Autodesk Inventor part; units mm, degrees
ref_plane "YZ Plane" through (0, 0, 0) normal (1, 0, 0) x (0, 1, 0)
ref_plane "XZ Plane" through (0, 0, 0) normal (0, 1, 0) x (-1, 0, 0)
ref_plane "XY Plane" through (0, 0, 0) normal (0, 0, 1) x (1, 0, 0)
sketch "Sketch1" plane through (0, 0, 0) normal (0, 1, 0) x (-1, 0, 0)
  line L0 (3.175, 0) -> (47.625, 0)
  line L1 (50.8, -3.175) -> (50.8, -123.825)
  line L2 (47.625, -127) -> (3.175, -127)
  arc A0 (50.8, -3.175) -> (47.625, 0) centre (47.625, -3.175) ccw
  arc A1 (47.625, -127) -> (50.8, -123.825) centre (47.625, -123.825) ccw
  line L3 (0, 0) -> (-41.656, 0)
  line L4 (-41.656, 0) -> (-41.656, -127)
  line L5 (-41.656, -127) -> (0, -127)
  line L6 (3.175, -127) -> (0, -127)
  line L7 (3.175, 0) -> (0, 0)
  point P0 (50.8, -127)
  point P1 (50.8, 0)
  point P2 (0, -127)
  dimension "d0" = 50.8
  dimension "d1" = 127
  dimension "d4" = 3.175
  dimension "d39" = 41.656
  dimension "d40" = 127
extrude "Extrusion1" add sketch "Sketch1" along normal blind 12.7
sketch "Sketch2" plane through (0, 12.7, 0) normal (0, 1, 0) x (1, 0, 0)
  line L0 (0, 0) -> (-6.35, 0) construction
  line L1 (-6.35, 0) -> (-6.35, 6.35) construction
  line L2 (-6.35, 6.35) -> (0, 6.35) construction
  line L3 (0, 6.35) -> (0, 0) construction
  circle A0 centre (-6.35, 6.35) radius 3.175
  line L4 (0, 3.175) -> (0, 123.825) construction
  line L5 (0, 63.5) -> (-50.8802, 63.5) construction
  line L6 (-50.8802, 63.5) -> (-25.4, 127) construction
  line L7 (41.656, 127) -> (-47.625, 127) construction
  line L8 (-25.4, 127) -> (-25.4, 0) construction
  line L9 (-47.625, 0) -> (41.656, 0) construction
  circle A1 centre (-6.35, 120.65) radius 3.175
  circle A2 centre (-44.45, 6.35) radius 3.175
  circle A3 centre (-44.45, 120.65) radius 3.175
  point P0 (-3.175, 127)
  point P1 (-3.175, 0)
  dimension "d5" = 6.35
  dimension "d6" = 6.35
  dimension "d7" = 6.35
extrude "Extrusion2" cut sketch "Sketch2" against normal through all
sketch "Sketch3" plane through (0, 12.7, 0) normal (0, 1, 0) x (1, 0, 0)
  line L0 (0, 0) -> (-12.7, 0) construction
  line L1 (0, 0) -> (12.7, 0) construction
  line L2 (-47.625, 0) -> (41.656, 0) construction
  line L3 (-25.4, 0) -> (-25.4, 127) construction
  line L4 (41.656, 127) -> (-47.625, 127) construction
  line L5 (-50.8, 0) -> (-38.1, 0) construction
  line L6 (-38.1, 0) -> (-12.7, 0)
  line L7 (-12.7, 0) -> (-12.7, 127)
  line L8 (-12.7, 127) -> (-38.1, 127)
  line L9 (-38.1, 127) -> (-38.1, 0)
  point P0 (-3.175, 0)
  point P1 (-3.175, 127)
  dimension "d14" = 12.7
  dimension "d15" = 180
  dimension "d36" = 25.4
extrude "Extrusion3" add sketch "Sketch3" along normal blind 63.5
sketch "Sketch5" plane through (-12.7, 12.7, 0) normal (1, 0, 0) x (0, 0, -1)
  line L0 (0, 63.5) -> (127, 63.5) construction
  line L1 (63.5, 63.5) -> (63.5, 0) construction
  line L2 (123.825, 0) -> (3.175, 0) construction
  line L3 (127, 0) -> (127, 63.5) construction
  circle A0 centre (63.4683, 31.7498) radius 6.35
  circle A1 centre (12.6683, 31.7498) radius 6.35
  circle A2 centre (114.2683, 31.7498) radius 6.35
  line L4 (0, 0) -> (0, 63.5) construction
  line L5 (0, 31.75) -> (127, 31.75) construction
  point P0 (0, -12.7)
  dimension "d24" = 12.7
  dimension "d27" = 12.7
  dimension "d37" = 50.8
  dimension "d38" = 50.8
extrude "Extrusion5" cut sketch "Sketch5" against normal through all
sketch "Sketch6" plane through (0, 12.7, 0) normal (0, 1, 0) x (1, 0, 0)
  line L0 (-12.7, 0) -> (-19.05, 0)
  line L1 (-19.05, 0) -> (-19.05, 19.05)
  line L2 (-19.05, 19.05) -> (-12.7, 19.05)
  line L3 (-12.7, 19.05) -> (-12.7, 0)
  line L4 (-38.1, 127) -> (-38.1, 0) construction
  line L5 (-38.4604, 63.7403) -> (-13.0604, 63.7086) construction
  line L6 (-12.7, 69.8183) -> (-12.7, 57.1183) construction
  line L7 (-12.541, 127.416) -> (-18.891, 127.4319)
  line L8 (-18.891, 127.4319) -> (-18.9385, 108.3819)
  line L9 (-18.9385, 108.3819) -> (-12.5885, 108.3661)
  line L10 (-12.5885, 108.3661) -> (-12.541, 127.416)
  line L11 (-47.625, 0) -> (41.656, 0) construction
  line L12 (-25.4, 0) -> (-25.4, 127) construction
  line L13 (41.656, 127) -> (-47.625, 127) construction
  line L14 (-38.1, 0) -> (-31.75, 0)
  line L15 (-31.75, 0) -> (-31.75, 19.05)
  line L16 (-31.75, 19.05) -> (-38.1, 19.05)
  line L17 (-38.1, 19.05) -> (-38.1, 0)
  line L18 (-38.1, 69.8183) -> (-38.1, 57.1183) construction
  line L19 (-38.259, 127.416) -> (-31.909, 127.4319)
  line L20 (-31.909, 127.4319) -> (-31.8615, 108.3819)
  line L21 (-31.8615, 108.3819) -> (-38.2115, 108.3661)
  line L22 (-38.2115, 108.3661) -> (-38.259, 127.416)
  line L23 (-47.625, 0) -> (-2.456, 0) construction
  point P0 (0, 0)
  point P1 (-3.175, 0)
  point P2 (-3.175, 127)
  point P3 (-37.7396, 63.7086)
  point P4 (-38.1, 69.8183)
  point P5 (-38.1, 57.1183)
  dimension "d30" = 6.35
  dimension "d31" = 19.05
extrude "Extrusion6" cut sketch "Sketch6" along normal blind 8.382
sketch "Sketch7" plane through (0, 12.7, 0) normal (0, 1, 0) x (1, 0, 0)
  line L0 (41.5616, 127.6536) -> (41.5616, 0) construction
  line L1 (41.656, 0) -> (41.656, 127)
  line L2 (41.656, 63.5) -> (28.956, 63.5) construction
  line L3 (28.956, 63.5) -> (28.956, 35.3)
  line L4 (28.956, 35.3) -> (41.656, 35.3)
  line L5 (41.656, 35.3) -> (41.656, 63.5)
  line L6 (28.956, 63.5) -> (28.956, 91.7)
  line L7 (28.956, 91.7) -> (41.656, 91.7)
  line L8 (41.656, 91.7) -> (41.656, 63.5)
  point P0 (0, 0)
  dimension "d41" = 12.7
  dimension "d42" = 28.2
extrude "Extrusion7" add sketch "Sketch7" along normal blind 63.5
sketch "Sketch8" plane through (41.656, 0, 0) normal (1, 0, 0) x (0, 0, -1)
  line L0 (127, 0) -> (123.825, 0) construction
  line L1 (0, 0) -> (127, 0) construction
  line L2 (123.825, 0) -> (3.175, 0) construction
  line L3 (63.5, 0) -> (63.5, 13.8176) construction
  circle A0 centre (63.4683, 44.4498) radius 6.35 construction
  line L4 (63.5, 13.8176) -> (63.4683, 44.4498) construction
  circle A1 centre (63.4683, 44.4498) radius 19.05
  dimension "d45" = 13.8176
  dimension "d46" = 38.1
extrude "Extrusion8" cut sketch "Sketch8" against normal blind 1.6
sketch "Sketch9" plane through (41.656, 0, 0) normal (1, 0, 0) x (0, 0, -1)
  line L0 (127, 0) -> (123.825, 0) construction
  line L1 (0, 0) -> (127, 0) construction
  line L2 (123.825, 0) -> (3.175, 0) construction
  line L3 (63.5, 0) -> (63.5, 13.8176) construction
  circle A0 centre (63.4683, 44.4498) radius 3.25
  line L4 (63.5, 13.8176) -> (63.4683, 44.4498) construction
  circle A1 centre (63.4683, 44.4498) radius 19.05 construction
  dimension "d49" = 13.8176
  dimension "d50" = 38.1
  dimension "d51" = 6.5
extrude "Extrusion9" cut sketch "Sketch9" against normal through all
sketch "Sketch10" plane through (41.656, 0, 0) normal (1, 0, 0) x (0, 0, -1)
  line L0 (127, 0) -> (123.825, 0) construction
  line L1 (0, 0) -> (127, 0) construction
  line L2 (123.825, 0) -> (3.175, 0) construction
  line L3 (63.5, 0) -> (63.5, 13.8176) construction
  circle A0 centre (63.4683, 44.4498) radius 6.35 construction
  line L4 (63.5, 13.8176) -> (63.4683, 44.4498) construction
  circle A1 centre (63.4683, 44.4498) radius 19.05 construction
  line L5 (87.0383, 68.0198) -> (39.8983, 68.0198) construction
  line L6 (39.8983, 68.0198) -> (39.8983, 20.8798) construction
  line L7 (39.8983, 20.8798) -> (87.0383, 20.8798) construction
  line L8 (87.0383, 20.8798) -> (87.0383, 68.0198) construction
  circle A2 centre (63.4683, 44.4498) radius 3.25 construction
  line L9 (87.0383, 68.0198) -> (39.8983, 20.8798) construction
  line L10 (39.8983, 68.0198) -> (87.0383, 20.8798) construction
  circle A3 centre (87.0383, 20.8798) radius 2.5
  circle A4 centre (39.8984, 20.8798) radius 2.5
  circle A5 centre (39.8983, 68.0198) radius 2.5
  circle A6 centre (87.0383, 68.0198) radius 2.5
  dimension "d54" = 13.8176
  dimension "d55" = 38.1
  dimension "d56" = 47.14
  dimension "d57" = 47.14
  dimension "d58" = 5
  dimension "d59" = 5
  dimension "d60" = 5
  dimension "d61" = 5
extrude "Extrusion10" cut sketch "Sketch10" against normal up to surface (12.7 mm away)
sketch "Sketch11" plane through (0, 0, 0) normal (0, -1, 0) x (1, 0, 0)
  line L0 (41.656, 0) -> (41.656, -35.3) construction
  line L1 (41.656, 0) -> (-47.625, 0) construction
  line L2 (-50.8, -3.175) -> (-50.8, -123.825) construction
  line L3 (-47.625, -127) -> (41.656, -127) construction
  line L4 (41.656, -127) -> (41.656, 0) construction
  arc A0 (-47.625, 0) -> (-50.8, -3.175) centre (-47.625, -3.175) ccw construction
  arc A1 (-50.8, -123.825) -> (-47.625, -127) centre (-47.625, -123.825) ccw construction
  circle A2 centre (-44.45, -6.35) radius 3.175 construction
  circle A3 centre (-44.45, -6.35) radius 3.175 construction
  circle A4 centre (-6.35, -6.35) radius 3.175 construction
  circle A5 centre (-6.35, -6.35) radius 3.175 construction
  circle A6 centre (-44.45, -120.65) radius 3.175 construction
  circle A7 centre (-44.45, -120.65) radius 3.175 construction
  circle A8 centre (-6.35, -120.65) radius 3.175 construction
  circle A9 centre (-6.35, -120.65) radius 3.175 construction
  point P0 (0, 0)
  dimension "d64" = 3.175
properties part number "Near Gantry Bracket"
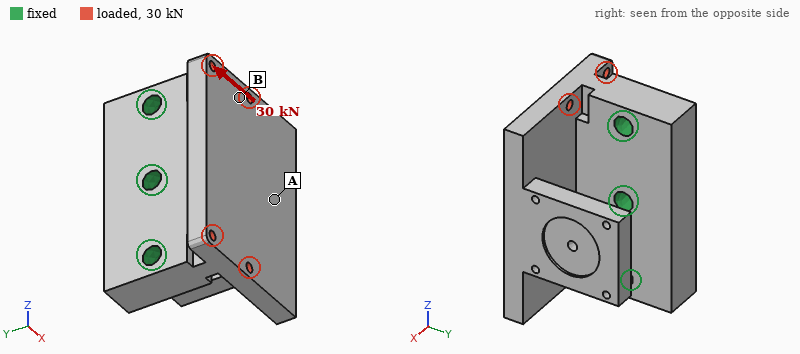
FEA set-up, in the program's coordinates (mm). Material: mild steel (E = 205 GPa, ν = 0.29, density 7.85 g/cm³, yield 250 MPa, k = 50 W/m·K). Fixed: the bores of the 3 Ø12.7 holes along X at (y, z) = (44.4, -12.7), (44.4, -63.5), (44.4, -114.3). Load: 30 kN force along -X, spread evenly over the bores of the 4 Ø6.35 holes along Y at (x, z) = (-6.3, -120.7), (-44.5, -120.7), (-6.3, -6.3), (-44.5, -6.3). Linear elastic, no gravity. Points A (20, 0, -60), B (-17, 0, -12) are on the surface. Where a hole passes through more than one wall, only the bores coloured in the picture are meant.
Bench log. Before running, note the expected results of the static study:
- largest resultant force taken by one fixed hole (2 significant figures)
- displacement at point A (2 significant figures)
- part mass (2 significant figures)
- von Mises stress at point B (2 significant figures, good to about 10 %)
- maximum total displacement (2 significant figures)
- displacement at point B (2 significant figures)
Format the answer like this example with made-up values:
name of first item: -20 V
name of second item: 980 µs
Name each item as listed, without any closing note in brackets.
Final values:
largest resultant force taken by one fixed hole: 10 kN
displacement at point A: 41 µm
part mass: 3.0 kg
von Mises stress at point B: 34 MPa
maximum total displacement: 58 µm
displacement at point B: 31 µm
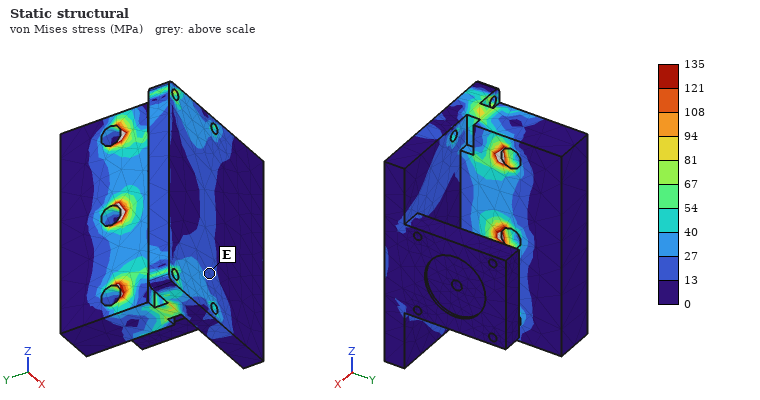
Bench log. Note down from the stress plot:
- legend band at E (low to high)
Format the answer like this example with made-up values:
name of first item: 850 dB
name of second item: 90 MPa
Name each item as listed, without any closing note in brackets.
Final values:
legend band at E: 13 to 27 MPa
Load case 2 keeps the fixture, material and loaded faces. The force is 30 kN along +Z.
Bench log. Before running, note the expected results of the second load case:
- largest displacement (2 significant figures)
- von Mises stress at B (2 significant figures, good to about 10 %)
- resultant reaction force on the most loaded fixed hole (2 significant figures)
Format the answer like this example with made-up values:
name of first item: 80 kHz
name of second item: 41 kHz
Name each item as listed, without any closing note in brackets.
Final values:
largest displacement: 13 µm
von Mises stress at B: 24 MPa
resultant reaction force on the most loaded fixed hole: 13 kN
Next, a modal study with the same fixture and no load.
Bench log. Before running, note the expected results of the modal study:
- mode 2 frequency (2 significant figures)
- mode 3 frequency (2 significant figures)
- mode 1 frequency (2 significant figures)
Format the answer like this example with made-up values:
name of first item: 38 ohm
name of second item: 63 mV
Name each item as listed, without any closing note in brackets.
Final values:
mode 2 frequency: 1900 Hz
mode 3 frequency: 2300 Hz
mode 1 frequency: 1200 Hz
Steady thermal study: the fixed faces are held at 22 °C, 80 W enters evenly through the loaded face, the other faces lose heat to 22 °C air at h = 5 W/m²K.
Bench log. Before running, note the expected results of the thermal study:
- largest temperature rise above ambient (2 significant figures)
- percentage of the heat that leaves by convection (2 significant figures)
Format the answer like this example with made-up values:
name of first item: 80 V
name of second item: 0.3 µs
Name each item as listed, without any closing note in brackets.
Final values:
largest temperature rise above ambient: 50 K
percentage of the heat that leaves by convection: 5.6 %
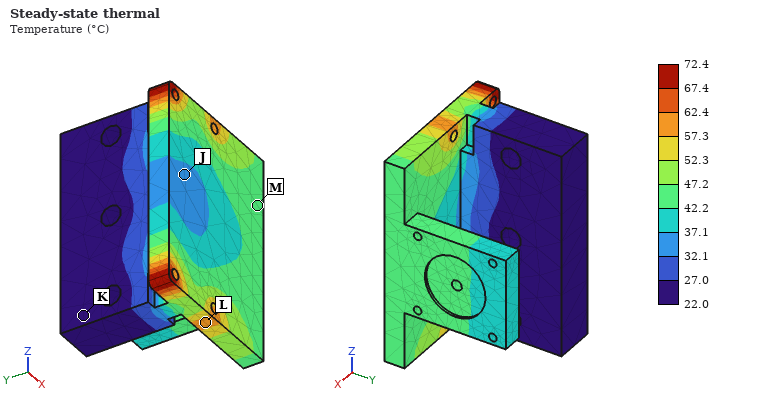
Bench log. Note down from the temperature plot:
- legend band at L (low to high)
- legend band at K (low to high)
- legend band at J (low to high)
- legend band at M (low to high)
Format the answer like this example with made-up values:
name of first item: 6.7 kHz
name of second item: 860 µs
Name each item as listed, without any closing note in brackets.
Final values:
legend band at L: 57.3 to 62.4 °C
legend band at K: 22.0 to 27.0 °C
legend band at J: 32.1 to 37.1 °C
legend band at M: 42.2 to 47.2 °C
